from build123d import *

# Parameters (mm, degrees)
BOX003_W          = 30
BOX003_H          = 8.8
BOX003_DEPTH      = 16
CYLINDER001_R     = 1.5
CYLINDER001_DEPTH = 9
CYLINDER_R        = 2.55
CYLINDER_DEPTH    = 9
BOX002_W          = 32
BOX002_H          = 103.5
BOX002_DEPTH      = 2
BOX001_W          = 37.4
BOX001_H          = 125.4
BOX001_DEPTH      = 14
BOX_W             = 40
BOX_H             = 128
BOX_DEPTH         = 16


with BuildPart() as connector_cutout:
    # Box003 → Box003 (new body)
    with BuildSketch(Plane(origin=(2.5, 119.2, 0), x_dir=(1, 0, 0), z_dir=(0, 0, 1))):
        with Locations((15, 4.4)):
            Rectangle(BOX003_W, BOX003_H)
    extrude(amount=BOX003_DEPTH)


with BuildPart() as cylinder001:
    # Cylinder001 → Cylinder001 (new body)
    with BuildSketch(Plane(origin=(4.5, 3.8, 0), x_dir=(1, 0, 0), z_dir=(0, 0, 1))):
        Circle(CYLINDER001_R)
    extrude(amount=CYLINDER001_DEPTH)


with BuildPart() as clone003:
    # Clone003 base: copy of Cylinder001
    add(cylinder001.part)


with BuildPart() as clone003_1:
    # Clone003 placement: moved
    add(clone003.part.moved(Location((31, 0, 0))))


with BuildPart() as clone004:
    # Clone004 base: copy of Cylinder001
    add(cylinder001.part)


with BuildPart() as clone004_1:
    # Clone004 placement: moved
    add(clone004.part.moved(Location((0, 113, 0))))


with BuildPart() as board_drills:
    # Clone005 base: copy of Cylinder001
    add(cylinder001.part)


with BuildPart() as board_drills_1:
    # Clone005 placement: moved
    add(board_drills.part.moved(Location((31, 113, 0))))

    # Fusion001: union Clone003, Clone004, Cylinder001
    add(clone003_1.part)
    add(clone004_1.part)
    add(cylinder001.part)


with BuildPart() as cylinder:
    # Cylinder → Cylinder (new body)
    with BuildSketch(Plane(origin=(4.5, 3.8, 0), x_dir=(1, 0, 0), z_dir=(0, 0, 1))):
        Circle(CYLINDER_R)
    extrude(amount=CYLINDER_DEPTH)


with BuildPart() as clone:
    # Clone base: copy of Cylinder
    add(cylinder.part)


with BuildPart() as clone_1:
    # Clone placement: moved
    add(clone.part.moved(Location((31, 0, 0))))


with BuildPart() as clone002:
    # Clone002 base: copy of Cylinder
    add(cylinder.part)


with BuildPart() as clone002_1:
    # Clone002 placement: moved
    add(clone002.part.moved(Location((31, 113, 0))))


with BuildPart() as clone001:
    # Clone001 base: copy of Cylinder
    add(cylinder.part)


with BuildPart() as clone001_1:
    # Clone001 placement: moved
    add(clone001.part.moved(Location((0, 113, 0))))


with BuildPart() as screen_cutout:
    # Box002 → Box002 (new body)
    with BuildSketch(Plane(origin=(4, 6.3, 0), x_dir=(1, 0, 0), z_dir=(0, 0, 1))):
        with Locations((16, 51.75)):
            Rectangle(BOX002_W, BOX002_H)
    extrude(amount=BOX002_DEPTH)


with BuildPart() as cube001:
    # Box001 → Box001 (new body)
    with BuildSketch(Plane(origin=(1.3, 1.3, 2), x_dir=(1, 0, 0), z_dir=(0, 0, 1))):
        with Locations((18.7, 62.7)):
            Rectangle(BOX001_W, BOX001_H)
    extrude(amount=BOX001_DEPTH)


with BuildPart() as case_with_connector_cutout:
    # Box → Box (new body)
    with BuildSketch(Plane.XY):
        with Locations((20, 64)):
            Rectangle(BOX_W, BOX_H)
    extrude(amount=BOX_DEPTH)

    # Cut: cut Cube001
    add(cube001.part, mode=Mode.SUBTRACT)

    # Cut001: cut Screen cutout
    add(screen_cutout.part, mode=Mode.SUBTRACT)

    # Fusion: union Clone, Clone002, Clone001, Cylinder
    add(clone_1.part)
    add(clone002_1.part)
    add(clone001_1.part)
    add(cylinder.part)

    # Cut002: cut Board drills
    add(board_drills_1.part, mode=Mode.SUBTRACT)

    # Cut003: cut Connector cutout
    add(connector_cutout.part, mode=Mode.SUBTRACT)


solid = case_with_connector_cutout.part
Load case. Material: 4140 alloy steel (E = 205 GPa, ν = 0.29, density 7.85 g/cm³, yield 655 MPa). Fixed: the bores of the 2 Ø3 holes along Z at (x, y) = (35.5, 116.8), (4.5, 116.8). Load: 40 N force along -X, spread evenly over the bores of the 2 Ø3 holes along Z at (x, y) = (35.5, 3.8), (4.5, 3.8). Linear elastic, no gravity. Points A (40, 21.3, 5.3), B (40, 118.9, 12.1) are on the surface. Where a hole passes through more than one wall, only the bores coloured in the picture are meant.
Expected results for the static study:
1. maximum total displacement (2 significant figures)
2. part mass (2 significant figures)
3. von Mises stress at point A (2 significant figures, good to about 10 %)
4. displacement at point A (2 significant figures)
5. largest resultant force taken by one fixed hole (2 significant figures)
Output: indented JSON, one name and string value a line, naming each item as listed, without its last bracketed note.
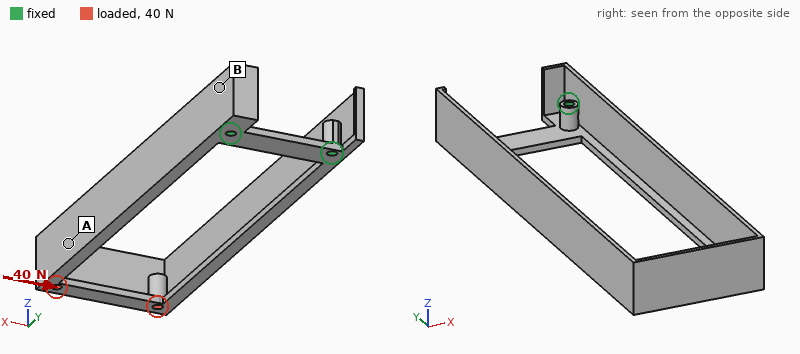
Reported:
{
  "maximum total displacement": "0.71 mm",
  "part mass": "70 g",
  "von Mises stress at point A": "44 MPa",
  "displacement at point A": "0.60 mm",
  "largest resultant force taken by one fixed hole": "100 N"
}
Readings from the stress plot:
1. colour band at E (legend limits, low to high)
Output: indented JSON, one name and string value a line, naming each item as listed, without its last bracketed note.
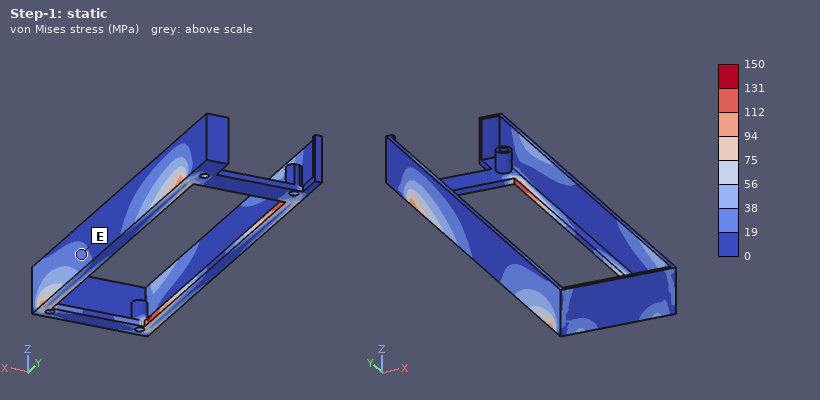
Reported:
{
  "colour band at E": "19 to 38 MPa"
}
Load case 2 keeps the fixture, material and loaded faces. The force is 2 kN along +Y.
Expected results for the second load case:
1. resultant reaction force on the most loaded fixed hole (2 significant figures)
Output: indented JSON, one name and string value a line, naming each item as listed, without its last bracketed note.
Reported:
{
  "resultant reaction force on the most loaded fixed hole": "1.0 kN"
}
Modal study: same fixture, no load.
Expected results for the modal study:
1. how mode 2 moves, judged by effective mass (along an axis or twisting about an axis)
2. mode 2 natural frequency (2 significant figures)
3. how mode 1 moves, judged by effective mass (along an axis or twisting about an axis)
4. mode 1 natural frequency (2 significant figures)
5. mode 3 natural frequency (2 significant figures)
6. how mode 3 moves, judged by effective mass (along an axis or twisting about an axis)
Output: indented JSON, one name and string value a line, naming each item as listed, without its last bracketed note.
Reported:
{
  "how mode 2 moves, judged by effective mass": "along Z",
  "mode 2 natural frequency": "350 Hz",
  "how mode 1 moves, judged by effective mass": "along X",
  "mode 1 natural frequency": "230 Hz",
  "mode 3 natural frequency": "540 Hz",
  "how mode 3 moves, judged by effective mass": "twisting about Y"
}
